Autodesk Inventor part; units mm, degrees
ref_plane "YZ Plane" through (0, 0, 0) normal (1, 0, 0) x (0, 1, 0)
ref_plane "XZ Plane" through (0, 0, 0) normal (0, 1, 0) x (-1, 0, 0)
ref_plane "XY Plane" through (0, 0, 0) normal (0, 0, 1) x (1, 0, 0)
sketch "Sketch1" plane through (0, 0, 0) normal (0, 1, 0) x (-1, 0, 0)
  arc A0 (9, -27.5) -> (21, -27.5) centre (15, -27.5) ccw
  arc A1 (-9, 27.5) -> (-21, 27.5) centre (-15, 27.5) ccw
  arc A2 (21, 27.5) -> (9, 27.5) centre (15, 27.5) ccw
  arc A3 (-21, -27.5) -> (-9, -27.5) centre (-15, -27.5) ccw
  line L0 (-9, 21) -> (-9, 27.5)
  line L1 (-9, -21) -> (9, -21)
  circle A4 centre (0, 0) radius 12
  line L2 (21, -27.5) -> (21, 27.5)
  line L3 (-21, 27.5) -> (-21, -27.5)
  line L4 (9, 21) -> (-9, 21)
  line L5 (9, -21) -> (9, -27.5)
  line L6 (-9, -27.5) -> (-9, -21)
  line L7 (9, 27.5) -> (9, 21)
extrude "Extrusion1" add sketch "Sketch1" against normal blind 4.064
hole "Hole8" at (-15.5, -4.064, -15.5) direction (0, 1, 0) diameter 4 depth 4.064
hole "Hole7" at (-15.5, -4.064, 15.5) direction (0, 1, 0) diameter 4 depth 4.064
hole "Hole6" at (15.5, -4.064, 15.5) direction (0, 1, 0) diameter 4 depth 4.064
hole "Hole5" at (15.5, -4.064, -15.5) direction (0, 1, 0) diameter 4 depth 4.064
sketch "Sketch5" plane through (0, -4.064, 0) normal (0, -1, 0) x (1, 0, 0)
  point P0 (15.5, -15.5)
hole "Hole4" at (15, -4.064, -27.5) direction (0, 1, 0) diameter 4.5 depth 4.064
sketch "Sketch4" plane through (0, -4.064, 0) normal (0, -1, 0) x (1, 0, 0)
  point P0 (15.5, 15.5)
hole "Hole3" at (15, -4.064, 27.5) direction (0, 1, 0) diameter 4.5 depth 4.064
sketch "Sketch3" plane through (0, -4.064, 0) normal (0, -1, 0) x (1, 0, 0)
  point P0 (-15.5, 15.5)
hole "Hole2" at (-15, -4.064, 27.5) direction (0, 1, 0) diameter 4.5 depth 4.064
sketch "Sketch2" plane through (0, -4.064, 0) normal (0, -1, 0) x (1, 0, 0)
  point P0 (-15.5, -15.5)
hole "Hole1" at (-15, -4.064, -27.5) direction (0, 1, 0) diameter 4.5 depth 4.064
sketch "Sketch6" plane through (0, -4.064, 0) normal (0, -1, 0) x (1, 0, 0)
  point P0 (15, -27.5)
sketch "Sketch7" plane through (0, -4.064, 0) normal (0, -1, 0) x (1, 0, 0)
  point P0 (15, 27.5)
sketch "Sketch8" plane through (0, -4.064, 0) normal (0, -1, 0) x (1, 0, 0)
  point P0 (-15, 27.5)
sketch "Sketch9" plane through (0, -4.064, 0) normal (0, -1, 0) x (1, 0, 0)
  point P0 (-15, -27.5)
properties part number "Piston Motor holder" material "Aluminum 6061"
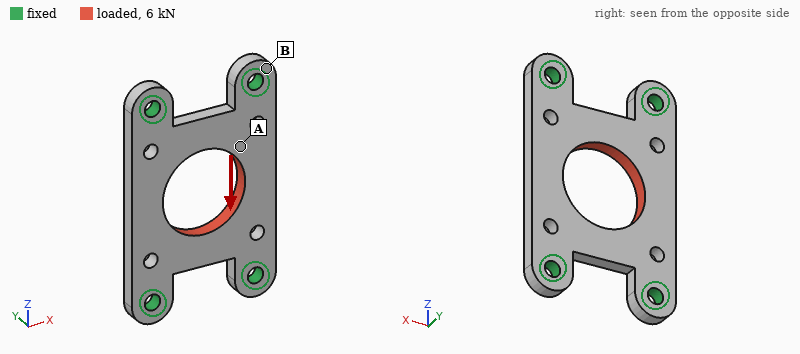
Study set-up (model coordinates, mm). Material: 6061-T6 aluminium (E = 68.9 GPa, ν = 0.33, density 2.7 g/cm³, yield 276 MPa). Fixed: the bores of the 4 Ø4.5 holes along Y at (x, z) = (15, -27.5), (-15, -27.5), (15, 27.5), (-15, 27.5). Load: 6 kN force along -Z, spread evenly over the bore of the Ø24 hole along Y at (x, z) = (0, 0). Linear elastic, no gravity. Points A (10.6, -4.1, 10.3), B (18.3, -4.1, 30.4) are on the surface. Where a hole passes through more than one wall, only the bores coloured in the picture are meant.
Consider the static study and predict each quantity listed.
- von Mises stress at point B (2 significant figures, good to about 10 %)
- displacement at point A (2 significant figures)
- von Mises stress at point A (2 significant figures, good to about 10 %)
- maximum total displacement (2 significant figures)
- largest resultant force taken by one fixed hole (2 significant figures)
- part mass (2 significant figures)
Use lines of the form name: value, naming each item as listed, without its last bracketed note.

von Mises stress at point B: 9.7 MPa
displacement at point A: 8.7 µm
von Mises stress at point A: 30 MPa
maximum total displacement: 13 µm
largest resultant force taken by one fixed hole: 1.6 kN
part mass: 19 g
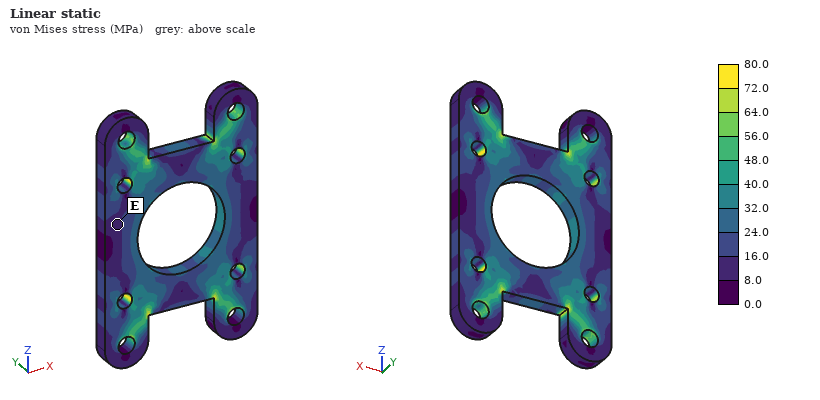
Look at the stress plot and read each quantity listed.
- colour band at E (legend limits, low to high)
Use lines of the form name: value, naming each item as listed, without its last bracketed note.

colour band at E: 8.0 to 16.0 MPa
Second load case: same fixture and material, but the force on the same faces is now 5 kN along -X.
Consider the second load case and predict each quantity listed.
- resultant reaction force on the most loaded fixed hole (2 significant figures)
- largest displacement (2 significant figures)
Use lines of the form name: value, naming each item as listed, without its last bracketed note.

resultant reaction force on the most loaded fixed hole: 1.4 kN
largest displacement: 37 µm
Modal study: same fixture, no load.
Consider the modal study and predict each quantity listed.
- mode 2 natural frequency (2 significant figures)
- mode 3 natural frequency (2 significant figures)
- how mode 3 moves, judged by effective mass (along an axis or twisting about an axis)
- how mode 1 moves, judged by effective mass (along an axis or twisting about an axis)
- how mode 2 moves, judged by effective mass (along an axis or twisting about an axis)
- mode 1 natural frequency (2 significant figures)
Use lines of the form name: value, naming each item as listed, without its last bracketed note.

mode 2 natural frequency: 8600 Hz
mode 3 natural frequency: 14 kHz
how mode 3 moves, judged by effective mass: twisting about X
how mode 1 moves, judged by effective mass: along Y
how mode 2 moves, judged by effective mass: twisting about Z
mode 1 natural frequency: 7000 Hz
